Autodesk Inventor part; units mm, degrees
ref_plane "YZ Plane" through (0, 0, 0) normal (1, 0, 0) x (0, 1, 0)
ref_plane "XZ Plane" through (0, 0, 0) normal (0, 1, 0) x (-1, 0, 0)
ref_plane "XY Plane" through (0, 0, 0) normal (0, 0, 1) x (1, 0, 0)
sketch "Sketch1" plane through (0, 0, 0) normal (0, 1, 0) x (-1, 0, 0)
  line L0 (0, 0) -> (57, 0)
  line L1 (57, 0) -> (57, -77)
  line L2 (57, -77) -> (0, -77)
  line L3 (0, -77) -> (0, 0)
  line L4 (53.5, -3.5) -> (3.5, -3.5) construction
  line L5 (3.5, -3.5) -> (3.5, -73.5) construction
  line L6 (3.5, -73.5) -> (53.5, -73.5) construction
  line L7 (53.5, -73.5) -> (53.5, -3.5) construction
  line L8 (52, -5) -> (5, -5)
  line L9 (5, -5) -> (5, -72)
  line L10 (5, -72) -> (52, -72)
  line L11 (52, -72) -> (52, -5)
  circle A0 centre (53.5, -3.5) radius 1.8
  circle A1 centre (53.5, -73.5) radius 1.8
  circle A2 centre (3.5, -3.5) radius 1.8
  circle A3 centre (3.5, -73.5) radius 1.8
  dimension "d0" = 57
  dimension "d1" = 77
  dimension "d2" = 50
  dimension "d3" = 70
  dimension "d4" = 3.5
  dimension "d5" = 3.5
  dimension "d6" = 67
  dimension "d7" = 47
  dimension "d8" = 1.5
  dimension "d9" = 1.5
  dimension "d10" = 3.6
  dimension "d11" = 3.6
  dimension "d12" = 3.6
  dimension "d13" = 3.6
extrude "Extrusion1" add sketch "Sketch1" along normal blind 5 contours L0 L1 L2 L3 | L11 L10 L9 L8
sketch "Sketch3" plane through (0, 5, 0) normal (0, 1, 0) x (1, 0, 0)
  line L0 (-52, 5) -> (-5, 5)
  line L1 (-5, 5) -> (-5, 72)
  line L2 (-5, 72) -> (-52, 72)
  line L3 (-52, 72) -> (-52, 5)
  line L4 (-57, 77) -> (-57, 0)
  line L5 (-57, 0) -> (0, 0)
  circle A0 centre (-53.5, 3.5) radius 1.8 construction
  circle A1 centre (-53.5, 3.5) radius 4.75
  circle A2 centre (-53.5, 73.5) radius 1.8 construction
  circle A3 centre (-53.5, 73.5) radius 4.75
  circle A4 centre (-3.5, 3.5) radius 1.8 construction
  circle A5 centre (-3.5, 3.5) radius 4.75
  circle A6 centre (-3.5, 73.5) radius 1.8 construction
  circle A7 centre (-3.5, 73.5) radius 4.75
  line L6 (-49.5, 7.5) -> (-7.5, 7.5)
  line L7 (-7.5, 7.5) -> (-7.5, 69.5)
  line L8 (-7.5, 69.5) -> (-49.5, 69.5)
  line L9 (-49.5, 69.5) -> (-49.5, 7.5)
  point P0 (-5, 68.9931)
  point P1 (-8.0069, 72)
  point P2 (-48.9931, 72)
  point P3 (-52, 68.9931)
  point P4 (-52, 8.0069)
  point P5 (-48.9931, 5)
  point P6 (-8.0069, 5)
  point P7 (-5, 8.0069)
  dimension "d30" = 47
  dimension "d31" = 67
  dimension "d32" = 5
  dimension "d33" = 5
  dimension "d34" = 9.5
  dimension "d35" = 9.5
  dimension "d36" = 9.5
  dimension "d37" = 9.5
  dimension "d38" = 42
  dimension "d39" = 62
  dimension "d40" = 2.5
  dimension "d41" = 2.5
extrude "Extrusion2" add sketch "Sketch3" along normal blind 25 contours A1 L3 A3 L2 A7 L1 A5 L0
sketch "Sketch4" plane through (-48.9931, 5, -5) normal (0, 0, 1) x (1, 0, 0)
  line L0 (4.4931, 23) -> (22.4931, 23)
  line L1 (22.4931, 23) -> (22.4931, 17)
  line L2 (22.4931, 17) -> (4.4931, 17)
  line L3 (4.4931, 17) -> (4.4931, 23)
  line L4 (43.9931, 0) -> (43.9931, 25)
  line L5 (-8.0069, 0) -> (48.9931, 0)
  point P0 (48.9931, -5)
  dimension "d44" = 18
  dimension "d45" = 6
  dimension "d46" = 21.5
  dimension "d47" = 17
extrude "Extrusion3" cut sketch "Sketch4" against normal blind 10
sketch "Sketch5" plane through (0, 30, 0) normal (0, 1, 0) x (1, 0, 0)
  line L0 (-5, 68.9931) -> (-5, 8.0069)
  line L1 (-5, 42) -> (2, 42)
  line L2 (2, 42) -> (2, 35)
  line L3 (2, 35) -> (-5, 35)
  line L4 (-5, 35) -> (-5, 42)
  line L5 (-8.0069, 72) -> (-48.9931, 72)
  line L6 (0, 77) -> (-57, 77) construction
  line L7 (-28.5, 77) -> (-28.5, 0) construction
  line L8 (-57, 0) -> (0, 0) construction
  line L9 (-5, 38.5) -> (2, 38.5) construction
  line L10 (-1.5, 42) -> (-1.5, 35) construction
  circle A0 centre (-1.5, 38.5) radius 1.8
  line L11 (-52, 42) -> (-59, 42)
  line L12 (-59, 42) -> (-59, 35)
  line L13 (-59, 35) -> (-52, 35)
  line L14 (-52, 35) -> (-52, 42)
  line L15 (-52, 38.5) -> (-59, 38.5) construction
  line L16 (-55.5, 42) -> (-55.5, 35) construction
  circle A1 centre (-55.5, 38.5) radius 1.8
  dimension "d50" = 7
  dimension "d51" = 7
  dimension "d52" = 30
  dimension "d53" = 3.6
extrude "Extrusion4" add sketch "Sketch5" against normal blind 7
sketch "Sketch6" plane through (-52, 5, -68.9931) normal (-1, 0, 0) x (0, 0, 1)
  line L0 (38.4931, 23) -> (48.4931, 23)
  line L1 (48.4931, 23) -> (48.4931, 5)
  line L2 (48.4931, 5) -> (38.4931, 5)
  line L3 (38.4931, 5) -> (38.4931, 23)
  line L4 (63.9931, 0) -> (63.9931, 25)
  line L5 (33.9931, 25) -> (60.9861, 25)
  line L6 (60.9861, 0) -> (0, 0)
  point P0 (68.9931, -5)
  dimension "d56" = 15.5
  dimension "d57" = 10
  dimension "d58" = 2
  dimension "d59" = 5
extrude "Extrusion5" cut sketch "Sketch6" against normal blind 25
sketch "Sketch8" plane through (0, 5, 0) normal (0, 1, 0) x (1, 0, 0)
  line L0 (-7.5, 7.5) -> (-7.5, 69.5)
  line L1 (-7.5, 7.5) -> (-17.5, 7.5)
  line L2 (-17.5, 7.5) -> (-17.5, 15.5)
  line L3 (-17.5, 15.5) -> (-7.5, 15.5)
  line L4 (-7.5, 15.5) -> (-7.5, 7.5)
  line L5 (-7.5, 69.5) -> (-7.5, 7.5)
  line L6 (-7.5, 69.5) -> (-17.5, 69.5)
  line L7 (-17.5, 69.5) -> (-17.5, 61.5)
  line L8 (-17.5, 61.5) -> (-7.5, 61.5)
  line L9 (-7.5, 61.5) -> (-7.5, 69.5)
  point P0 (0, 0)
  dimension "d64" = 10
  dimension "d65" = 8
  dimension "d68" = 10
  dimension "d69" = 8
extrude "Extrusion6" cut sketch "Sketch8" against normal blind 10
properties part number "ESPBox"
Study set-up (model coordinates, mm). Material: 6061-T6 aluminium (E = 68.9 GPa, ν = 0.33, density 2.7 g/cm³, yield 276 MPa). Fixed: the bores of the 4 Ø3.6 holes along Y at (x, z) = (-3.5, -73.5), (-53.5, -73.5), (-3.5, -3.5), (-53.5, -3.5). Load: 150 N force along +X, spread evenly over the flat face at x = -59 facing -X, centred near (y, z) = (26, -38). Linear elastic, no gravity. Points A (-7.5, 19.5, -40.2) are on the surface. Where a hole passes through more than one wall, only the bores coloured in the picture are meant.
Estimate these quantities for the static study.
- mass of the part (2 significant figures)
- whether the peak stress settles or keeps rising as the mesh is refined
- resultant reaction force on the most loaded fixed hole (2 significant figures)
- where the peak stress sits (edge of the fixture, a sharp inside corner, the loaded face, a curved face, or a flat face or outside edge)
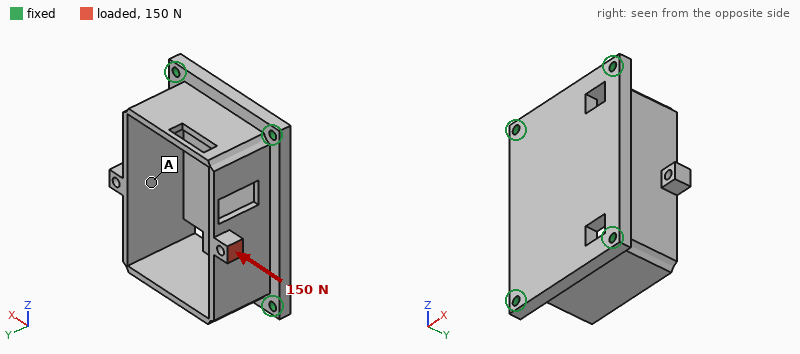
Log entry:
91 g
keeps rising
67 N
a sharp inside corner
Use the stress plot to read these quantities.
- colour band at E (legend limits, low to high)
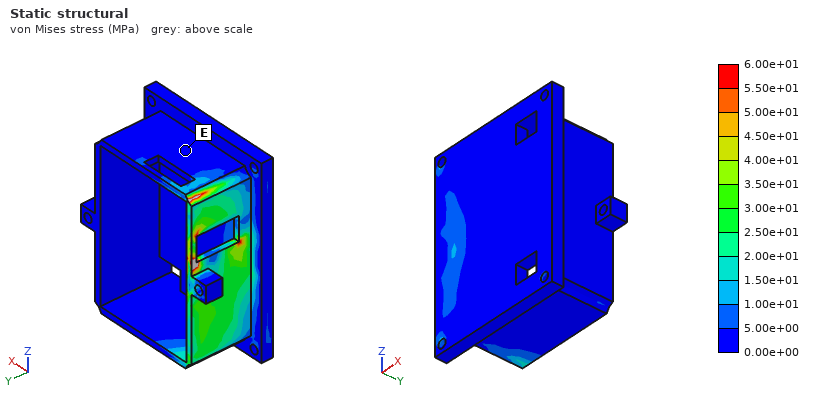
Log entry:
0.00e+00 to 5.00e+00 MPa
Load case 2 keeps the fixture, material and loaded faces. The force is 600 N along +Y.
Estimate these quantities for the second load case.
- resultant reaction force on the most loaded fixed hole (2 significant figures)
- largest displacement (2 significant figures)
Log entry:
400 N
0.43 mm
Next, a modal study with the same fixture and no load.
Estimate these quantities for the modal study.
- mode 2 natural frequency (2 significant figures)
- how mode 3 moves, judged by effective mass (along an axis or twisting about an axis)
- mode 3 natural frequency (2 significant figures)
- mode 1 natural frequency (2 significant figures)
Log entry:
3800 Hz
along Y
5900 Hz
3600 Hz
